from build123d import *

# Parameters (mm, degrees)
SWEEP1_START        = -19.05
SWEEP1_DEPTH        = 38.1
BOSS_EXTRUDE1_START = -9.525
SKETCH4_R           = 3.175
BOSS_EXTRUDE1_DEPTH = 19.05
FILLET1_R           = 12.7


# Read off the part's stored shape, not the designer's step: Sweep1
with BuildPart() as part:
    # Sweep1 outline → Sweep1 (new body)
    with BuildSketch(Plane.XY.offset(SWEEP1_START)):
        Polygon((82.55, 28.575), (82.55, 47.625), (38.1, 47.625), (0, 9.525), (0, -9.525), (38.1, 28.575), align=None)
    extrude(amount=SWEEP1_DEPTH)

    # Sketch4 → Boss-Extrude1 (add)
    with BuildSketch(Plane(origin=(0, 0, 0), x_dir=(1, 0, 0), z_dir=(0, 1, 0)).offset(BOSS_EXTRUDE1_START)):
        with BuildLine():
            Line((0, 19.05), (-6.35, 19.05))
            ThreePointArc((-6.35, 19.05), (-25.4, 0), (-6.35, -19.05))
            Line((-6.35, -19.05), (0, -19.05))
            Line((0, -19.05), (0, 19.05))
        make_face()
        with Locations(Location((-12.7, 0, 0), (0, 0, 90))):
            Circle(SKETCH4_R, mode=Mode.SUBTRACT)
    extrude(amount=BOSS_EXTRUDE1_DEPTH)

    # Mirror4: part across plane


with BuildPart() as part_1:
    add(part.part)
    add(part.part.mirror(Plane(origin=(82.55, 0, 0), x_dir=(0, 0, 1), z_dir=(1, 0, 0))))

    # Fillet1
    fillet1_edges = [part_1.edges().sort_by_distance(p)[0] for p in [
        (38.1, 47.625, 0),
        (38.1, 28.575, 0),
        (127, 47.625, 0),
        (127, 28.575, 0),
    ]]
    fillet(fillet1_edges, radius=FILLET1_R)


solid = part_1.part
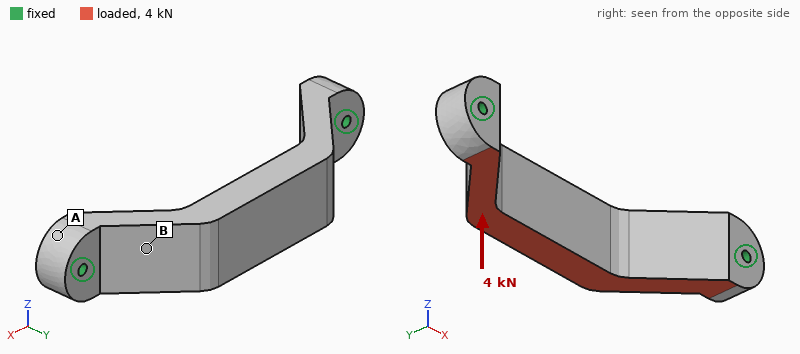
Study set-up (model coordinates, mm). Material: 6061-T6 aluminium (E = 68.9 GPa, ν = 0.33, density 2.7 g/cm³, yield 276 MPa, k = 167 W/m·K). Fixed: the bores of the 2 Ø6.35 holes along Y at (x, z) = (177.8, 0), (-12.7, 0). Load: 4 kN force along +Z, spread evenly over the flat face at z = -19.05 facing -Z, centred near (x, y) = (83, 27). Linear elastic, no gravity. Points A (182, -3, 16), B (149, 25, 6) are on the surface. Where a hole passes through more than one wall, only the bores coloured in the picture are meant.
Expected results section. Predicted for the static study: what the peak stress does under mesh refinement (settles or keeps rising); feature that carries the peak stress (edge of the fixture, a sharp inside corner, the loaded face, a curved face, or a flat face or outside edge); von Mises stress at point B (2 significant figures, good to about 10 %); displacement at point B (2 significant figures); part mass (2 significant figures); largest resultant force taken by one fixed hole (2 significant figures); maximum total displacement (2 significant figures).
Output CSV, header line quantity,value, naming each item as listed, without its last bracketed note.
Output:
quantity,value
what the peak stress does under mesh refinement,keeps rising
feature that carries the peak stress,edge of the fixture
von Mises stress at point B,21 MPa
displacement at point B,0.055 mm
part mass,400 g
largest resultant force taken by one fixed hole,2.0 kN
maximum total displacement,0.12 mm
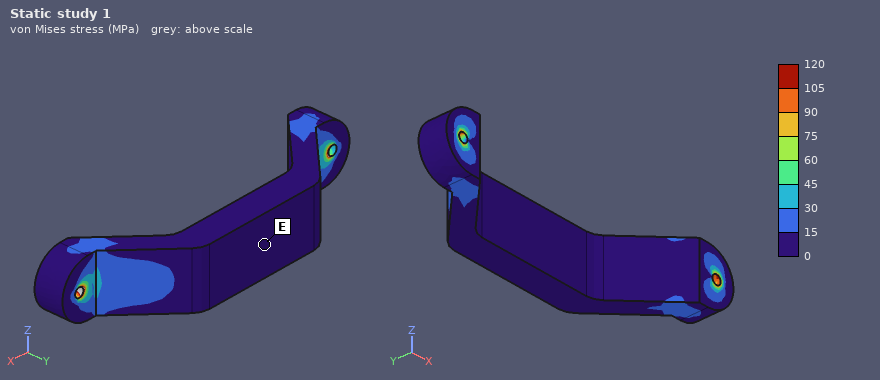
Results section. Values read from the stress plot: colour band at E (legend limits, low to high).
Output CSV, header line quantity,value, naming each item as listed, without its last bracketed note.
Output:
quantity,value
colour band at E,0 to 15 MPa
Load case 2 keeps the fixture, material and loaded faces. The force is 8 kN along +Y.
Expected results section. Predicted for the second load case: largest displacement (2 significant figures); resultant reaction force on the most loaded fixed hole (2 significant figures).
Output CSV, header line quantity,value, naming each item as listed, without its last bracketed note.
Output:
quantity,value
largest displacement,0.14 mm
resultant reaction force on the most loaded fixed hole,5.3 kN
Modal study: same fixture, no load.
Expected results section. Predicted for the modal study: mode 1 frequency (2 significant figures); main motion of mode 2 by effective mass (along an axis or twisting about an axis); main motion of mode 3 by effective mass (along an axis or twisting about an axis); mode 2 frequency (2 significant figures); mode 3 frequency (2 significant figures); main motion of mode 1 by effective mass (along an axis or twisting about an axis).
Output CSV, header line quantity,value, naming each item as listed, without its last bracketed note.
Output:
quantity,value
mode 1 frequency,1800 Hz
main motion of mode 2 by effective mass,along X
main motion of mode 3 by effective mass,along Y
mode 2 frequency,3700 Hz
mode 3 frequency,4600 Hz
main motion of mode 1 by effective mass,along Z
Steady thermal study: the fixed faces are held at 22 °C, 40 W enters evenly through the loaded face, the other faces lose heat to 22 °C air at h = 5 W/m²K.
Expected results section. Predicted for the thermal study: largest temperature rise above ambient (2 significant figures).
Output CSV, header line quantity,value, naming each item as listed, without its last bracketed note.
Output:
quantity,value
largest temperature rise above ambient,14 K
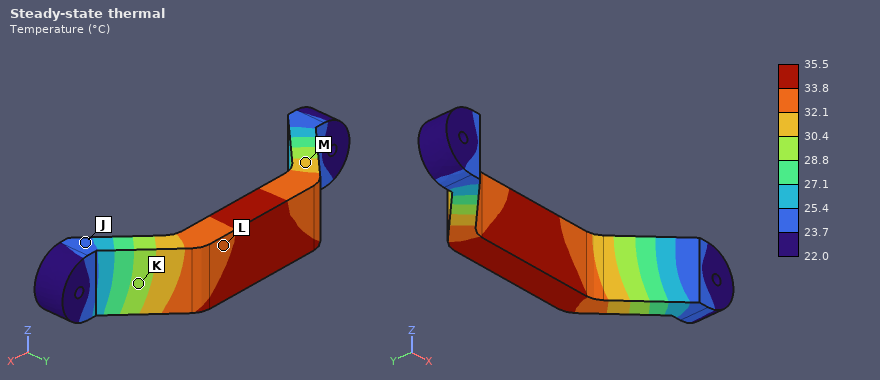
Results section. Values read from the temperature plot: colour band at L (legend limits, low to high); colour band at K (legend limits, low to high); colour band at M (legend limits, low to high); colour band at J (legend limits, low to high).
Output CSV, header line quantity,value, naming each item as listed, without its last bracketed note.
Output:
quantity,value
colour band at L,32.1 to 33.8 °C
colour band at K,28.8 to 30.4 °C
colour band at M,30.4 to 32.1 °C
colour band at J,23.7 to 25.4 °C
